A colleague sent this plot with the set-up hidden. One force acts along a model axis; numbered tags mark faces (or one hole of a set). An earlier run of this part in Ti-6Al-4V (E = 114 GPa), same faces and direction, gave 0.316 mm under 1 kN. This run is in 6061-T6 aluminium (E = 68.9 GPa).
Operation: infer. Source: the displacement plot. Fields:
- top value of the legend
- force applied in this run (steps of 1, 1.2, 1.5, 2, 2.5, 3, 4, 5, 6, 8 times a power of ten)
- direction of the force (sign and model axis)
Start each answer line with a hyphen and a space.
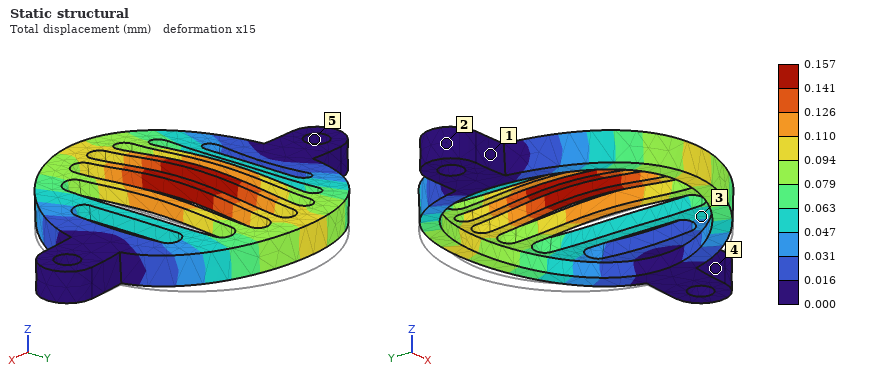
- 0.157 mm
- 300 N
- +Z
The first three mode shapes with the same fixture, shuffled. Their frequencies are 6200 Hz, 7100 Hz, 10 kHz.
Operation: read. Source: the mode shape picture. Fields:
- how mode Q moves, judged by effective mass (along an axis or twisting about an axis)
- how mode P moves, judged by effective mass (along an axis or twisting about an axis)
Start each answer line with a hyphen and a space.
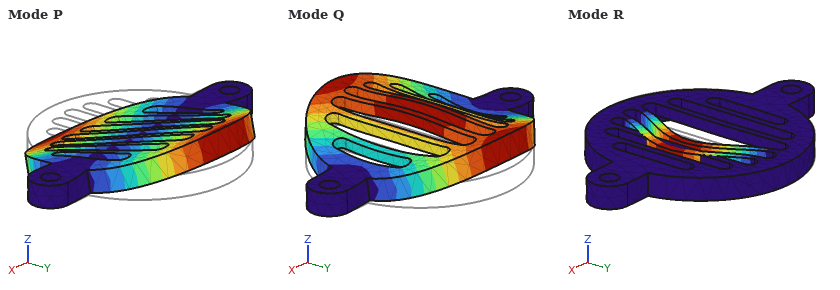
- along Z
- twisting about X
